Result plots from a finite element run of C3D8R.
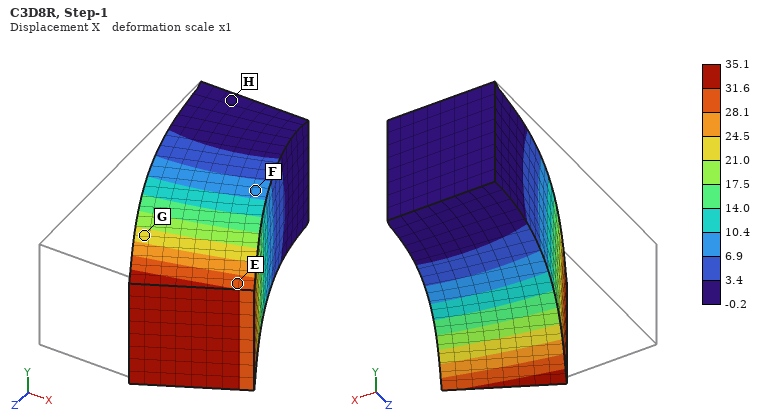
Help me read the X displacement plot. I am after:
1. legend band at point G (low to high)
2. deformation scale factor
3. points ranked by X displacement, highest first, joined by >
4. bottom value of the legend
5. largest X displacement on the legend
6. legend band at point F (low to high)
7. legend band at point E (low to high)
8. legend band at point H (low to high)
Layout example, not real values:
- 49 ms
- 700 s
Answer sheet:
- 21.0 to 24.5
- 1
- E > G > F > H
- -0.2
- 35.1
- 6.9 to 10.4
- 28.1 to 31.6
- -0.2 to 3.4
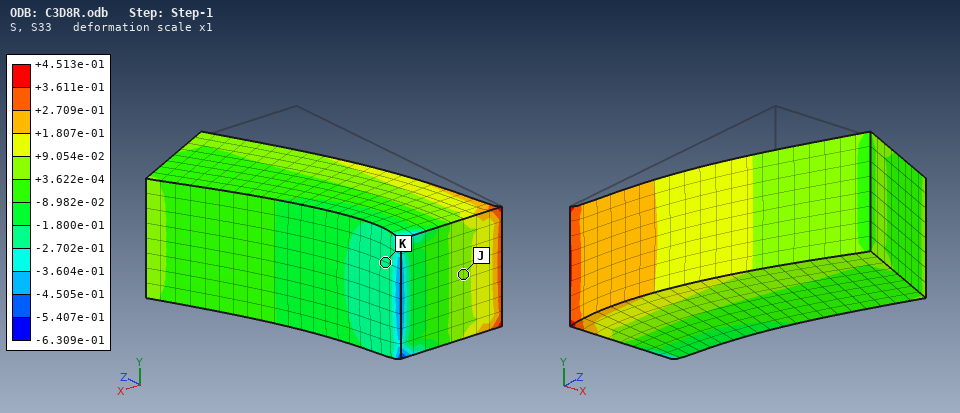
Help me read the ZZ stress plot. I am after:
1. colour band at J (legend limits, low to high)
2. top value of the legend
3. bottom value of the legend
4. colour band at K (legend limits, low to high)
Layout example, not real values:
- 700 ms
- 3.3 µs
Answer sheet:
- +3.622e-04 to +9.054e-02
- +4.513e-01
- -6.309e-01
- -2.702e-01 to -1.800e-01
